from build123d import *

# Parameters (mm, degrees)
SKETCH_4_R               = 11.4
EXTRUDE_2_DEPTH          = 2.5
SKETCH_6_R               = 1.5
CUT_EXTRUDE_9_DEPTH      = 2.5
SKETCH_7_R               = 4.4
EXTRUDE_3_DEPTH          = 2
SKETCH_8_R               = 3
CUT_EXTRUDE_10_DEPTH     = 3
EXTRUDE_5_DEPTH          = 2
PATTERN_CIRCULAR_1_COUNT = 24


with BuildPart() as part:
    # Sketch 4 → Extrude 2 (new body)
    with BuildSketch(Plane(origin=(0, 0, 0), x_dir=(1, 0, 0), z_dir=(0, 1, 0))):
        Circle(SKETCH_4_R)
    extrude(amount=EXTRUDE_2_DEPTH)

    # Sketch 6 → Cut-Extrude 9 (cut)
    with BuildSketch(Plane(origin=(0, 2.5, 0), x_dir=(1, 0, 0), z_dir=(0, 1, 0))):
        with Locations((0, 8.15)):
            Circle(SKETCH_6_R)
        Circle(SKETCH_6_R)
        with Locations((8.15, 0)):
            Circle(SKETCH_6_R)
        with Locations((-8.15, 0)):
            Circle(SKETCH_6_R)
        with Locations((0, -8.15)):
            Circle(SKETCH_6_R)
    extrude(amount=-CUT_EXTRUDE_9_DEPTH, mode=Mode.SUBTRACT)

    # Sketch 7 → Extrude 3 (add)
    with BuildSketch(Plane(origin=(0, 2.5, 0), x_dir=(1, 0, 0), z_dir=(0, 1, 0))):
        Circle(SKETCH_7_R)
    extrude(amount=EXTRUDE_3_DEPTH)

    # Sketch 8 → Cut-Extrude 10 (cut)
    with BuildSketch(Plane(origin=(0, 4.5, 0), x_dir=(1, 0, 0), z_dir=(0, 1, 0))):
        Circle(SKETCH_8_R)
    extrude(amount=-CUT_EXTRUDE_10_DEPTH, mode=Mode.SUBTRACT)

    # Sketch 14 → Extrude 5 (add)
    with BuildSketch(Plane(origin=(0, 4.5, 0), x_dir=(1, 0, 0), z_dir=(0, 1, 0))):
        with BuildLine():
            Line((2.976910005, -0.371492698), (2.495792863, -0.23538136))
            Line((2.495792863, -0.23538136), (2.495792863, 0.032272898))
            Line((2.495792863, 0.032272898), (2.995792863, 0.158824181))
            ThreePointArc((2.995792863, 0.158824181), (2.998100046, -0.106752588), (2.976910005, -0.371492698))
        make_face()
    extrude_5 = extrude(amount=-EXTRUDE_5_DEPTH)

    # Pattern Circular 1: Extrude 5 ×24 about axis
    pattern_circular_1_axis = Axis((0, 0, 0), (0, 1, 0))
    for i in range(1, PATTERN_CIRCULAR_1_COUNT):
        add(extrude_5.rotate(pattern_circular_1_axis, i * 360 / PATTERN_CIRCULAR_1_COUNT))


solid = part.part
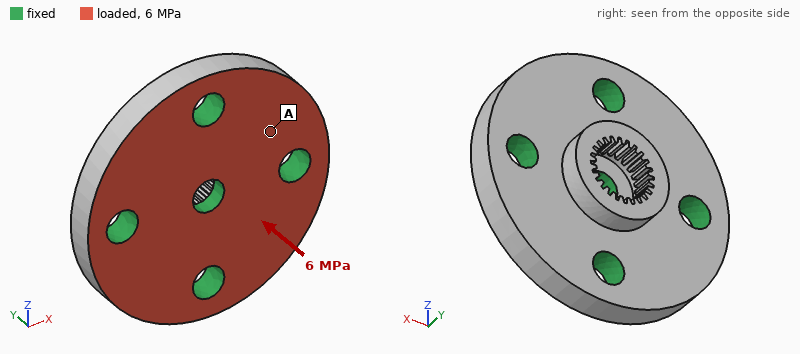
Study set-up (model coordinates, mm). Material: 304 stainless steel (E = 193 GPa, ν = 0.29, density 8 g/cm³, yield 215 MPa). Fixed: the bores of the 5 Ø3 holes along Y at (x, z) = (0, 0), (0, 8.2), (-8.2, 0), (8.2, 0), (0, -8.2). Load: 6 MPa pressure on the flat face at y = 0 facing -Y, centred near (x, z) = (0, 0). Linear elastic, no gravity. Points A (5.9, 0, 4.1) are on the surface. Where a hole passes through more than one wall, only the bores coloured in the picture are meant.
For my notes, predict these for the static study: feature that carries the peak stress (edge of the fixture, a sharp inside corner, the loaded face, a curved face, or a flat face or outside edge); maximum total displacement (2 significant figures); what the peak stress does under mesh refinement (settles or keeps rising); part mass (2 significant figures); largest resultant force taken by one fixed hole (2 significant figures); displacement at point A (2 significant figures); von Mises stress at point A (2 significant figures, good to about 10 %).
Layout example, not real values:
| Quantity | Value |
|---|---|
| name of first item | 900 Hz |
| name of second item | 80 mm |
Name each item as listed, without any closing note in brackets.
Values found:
| Quantity | Value |
|---|---|
| feature that carries the peak stress | edge of the fixture |
| maximum total displacement | 3.0 µm |
| what the peak stress does under mesh refinement | keeps rising |
| part mass | 7.9 g |
| largest resultant force taken by one fixed hole | 490 N |
| displacement at point A | 1.2 µm |
| von Mises stress at point A | 23 MPa |
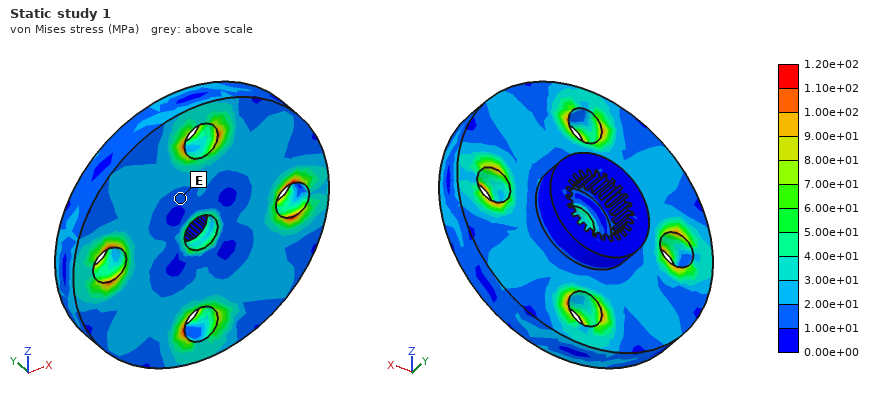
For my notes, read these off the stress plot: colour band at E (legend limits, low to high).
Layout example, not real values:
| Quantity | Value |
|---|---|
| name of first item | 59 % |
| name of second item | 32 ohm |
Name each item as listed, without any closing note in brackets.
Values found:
| Quantity | Value |
|---|---|
| colour band at E | 1.00e+01 to 2.00e+01 MPa |
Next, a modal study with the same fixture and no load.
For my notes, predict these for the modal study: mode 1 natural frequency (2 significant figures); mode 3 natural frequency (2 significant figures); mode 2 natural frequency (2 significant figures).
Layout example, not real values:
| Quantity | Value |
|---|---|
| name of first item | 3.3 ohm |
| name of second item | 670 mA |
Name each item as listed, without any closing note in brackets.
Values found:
| Quantity | Value |
|---|---|
| mode 1 natural frequency | 65 kHz |
| mode 3 natural frequency | 66 kHz |
| mode 2 natural frequency | 66 kHz |
